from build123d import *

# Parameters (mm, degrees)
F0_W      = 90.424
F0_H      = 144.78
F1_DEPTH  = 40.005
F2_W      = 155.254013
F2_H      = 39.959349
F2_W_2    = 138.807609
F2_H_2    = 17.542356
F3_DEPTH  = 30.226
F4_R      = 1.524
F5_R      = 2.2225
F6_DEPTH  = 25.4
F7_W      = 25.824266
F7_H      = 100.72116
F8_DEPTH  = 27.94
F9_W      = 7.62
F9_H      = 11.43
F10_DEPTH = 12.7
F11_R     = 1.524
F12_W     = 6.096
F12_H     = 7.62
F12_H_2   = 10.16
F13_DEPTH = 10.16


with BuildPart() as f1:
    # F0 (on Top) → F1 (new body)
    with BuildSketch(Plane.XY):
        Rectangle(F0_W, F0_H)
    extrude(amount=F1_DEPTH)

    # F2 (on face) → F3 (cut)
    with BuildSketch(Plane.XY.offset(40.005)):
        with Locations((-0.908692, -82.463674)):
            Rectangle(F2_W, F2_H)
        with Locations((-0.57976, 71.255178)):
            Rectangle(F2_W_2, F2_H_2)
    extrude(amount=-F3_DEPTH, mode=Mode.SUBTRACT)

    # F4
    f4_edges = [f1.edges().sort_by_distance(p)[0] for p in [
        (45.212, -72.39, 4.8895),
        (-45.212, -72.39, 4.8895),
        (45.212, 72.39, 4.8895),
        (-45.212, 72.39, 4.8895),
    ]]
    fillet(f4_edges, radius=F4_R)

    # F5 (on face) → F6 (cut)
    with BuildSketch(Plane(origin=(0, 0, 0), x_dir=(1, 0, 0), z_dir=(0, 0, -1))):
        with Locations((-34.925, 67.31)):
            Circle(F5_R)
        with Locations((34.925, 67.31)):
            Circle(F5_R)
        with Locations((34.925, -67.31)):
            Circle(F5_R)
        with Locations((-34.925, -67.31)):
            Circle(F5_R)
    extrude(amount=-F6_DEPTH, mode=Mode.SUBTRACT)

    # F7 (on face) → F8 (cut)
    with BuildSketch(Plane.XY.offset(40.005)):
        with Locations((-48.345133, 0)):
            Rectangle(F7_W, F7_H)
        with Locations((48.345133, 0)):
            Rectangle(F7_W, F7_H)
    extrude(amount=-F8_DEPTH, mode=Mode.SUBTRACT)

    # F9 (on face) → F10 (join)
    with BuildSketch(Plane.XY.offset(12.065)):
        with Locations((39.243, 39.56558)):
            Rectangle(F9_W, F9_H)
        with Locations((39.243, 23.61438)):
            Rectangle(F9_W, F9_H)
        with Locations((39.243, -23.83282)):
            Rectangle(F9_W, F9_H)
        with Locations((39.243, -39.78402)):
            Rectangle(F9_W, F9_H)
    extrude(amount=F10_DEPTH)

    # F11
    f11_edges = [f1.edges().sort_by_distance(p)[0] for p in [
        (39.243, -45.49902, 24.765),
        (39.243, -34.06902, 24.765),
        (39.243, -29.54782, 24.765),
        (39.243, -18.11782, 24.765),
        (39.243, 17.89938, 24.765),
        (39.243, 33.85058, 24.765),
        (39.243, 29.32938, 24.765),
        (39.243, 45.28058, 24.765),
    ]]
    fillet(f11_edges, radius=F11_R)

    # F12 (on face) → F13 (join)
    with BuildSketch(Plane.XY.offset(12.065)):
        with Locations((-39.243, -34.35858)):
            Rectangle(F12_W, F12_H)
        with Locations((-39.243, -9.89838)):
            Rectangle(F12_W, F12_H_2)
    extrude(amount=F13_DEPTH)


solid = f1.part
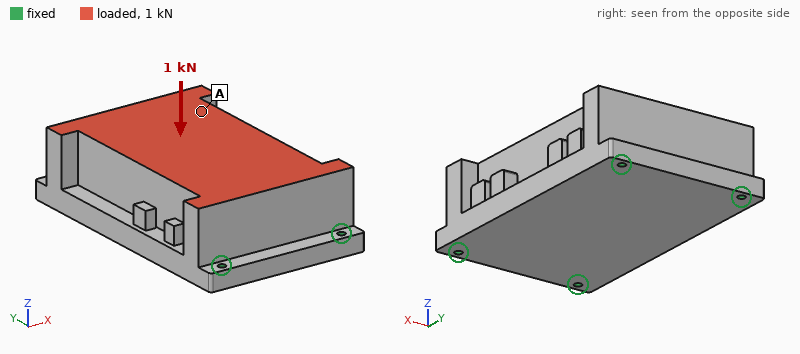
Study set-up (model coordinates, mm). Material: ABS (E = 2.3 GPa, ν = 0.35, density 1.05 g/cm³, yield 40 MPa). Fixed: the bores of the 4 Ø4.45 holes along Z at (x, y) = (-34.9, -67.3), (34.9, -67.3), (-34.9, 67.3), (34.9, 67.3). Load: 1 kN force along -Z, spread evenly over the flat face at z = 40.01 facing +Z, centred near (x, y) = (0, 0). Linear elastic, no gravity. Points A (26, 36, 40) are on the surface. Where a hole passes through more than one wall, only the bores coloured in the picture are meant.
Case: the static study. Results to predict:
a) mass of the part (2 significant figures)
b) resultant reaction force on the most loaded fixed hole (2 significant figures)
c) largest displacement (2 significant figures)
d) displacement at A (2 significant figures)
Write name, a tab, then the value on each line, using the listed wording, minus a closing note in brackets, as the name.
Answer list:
mass of the part	440 g
resultant reaction force on the most loaded fixed hole	300 N
largest displacement	51 µm
displacement at A	40 µm
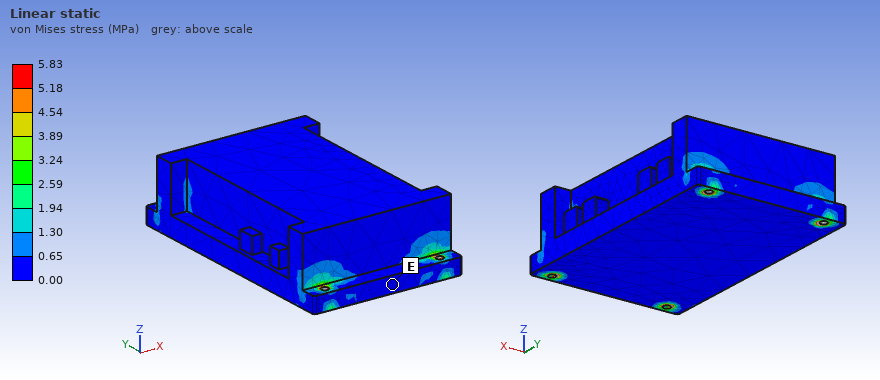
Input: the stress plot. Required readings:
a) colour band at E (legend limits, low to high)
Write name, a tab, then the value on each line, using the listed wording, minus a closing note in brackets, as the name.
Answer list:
colour band at E	0.00 to 0.65 MPa
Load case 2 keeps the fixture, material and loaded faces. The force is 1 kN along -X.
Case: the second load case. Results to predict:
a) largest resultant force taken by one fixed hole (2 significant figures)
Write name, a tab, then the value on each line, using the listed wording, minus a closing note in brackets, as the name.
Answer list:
largest resultant force taken by one fixed hole	390 N
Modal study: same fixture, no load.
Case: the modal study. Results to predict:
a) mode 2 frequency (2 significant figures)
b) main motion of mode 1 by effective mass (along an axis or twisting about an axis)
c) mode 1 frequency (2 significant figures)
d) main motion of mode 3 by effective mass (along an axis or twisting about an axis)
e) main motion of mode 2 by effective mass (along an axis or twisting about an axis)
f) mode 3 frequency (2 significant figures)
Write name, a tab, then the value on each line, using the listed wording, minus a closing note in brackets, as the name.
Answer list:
mode 2 frequency	1400 Hz
main motion of mode 1 by effective mass	along Z
mode 1 frequency	1200 Hz
main motion of mode 3 by effective mass	along X
main motion of mode 2 by effective mass	along X
mode 3 frequency	1900 Hz
